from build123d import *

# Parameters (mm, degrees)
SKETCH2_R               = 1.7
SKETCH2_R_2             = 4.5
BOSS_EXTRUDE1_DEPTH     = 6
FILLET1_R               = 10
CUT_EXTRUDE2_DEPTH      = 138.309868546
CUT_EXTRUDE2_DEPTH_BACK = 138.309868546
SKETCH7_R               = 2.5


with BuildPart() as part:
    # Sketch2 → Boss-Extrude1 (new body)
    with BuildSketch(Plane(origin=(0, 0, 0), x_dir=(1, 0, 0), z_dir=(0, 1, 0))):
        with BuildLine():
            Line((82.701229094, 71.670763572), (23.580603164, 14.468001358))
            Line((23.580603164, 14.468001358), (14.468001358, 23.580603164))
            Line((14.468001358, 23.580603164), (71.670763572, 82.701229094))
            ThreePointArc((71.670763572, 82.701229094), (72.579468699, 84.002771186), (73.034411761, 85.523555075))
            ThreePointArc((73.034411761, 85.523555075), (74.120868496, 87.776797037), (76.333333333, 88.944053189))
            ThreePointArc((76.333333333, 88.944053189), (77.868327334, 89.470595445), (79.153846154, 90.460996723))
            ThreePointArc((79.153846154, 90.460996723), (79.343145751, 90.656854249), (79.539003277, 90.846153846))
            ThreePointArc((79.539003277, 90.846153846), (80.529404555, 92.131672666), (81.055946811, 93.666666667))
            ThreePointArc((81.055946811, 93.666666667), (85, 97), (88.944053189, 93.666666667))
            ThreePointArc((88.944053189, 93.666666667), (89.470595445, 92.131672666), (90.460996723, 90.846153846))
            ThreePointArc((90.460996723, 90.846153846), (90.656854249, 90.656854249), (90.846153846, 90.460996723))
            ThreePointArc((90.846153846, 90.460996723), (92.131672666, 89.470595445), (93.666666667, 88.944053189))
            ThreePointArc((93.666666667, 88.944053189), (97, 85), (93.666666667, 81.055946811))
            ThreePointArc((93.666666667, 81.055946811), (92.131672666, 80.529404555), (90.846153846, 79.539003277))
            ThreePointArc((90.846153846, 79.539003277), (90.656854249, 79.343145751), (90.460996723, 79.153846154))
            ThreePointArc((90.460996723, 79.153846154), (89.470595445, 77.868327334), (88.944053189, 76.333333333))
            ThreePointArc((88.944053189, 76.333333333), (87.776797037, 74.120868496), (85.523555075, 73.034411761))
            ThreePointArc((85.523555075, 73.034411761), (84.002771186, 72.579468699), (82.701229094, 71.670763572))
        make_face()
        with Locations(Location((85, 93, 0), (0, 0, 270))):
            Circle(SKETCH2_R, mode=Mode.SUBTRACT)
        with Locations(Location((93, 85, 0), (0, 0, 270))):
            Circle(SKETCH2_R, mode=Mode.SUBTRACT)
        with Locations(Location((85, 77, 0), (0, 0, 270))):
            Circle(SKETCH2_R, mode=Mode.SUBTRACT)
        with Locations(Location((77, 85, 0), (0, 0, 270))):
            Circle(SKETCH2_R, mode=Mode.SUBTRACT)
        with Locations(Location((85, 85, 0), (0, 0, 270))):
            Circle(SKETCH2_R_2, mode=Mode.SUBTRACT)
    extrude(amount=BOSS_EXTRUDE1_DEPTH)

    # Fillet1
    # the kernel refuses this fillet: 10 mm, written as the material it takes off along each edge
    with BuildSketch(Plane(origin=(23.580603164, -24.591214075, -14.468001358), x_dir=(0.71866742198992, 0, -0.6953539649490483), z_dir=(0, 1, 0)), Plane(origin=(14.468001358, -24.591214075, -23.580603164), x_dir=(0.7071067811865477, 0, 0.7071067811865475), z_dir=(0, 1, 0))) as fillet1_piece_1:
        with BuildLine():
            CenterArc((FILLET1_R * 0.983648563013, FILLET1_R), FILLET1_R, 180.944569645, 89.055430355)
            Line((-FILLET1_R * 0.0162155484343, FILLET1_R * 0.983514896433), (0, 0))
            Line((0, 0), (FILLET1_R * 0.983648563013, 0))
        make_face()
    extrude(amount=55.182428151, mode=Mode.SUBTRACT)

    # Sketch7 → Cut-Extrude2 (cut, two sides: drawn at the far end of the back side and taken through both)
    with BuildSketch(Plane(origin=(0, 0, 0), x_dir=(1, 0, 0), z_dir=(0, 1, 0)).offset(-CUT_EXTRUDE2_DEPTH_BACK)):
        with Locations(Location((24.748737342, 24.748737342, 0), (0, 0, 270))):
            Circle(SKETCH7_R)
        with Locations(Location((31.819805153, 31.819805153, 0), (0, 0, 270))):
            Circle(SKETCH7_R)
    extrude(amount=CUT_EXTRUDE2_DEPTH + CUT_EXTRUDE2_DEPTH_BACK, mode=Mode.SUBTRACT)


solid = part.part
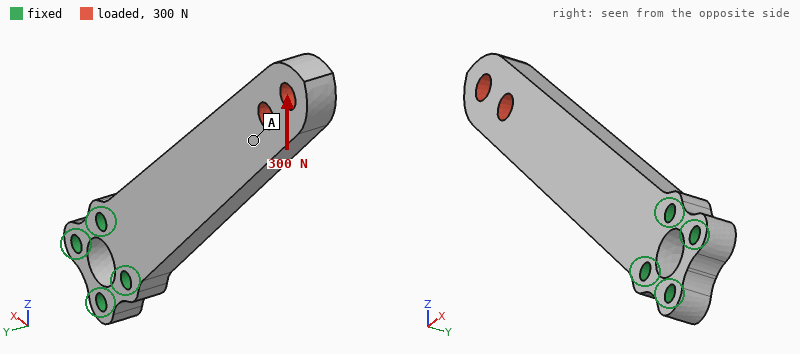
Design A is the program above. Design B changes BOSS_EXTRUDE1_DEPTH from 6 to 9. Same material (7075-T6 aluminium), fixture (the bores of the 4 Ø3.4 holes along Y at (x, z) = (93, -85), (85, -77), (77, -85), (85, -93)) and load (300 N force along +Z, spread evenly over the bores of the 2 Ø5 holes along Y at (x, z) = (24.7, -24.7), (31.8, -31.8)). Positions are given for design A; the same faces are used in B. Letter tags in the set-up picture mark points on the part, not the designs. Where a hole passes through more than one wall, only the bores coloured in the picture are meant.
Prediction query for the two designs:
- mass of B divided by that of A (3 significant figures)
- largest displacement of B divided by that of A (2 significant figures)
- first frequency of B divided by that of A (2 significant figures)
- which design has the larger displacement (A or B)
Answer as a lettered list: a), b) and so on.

a) 1.50
b) 0.67
c) 1.5
d) A
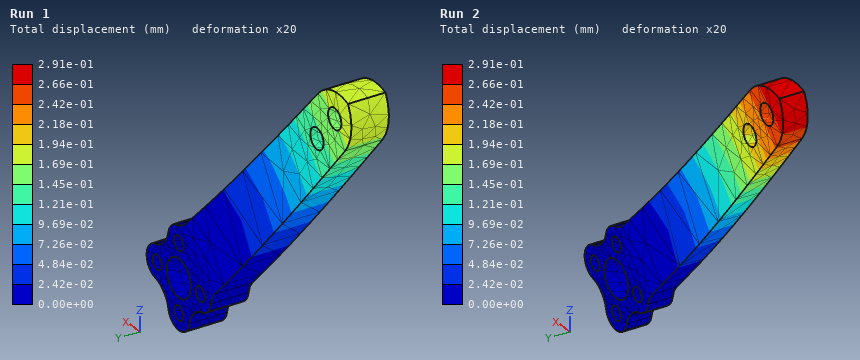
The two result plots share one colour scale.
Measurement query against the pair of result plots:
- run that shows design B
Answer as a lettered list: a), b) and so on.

a) Run 1
